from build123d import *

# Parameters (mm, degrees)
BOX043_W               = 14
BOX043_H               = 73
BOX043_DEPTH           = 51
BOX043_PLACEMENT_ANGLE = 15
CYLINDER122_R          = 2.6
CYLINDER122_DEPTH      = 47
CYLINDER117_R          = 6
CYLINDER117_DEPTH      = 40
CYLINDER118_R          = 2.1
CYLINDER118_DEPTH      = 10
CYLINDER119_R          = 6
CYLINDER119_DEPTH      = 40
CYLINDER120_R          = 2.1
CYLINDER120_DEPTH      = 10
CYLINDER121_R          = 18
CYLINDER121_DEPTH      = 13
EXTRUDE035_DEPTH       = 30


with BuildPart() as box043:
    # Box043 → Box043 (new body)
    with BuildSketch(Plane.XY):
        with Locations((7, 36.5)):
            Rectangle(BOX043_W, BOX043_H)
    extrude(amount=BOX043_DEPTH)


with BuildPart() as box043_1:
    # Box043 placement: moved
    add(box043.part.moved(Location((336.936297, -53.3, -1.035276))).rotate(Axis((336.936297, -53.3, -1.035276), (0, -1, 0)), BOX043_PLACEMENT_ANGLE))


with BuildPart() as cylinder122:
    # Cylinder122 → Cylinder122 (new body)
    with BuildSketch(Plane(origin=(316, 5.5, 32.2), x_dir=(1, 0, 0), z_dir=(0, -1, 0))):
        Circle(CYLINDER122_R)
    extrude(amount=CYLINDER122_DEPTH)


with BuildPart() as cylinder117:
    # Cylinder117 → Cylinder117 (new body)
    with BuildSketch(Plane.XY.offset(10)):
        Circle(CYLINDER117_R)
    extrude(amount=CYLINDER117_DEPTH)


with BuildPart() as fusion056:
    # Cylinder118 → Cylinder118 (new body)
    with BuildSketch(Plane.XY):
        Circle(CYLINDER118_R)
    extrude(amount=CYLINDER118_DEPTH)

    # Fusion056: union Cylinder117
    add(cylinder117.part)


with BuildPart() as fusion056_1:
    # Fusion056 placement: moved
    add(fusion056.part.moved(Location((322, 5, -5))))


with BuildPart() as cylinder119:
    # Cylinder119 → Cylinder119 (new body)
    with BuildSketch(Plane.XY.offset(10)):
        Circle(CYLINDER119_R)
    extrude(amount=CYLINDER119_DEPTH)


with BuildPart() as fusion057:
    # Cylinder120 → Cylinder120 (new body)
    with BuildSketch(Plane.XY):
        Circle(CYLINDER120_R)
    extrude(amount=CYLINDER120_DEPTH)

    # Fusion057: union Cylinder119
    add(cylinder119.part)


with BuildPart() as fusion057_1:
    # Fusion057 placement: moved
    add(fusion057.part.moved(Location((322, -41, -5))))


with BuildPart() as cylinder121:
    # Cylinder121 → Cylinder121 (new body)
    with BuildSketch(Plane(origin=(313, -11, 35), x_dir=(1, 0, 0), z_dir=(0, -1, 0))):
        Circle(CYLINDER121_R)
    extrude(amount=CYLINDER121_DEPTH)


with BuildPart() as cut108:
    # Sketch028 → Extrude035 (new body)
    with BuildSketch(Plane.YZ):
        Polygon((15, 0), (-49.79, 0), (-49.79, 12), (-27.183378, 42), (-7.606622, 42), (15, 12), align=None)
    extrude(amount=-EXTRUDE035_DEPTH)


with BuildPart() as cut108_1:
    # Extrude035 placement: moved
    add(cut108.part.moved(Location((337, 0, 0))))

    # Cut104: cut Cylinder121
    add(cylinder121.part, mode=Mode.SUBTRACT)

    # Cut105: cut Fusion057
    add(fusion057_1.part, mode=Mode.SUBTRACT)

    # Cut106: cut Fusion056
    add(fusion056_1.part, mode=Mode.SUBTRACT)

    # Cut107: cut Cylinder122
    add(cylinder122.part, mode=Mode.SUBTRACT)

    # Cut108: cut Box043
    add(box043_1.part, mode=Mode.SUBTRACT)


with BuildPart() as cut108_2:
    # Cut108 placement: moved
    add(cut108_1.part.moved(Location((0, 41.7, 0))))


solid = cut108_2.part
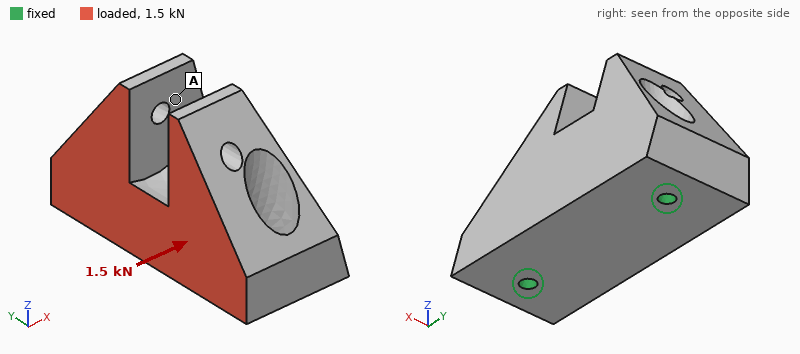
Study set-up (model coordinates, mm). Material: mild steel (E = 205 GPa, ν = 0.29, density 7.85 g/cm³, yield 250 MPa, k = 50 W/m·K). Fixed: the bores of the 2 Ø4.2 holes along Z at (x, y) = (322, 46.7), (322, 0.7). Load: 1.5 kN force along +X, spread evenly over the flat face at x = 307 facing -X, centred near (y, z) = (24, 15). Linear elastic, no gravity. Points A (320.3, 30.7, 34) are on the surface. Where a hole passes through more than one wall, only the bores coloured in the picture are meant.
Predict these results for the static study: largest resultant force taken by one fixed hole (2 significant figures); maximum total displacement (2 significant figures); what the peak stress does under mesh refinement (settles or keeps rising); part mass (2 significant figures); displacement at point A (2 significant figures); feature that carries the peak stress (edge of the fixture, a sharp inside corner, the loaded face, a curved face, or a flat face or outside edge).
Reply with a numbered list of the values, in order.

1. 770 N
2. 24 µm
3. keeps rising
4. 310 g
5. 18 µm
6. edge of the fixture
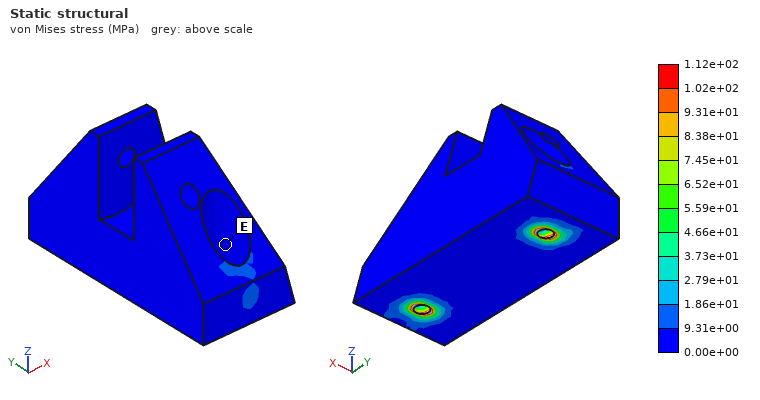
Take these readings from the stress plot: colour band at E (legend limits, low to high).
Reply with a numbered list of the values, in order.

1. 0.00e+00 to 9.31e+00 MPa
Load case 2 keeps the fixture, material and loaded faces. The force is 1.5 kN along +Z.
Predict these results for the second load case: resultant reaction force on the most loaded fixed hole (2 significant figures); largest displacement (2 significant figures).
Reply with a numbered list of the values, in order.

1. 800 N
2. 27 µm
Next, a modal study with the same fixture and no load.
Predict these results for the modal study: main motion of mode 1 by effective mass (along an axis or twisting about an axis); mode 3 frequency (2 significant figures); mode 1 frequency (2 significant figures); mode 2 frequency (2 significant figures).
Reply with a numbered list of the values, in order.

1. along X
2. 11 kHz
3. 3100 Hz
4. 11 kHz
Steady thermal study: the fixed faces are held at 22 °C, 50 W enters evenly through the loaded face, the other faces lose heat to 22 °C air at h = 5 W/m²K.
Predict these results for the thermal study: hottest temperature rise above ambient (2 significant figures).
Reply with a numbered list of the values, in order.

1. 44 K
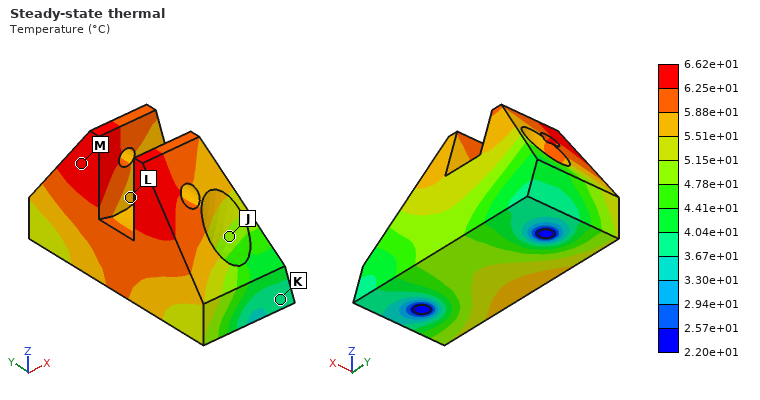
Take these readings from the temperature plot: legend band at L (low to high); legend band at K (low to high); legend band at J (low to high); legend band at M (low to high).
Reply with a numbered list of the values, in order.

1. 5.51e+01 to 5.88e+01 °C
2. 3.67e+01 to 4.04e+01 °C
3. 4.78e+01 to 5.15e+01 °C
4. 6.25e+01 to 6.62e+01 °C
